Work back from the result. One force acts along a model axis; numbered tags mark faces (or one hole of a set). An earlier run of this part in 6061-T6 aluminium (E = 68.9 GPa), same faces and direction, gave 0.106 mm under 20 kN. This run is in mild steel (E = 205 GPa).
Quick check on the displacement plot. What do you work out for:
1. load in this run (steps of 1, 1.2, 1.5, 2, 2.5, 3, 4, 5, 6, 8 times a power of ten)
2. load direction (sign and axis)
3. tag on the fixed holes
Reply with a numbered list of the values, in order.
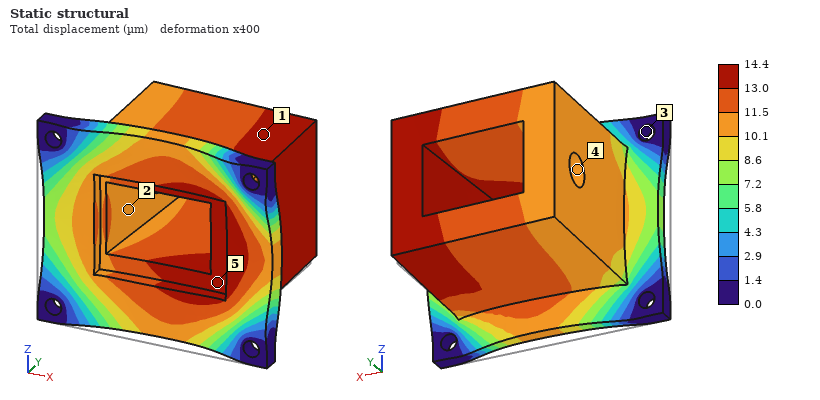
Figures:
1. 8 kN
2. +Y
3. 3
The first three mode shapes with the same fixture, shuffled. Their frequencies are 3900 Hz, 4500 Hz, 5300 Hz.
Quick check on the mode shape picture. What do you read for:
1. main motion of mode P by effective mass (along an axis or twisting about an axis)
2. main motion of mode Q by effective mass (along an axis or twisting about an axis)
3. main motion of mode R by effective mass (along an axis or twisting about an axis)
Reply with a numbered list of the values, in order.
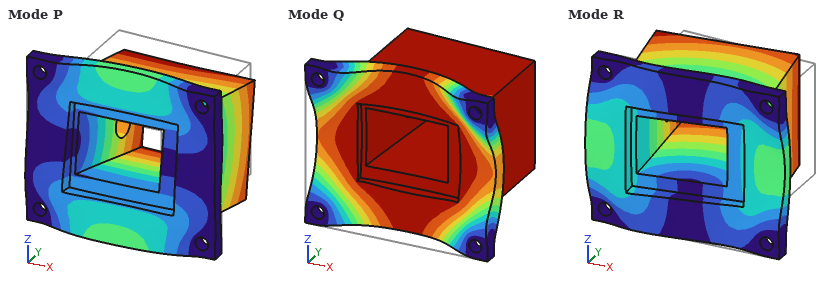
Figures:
1. along Z
2. along Y
3. along X
